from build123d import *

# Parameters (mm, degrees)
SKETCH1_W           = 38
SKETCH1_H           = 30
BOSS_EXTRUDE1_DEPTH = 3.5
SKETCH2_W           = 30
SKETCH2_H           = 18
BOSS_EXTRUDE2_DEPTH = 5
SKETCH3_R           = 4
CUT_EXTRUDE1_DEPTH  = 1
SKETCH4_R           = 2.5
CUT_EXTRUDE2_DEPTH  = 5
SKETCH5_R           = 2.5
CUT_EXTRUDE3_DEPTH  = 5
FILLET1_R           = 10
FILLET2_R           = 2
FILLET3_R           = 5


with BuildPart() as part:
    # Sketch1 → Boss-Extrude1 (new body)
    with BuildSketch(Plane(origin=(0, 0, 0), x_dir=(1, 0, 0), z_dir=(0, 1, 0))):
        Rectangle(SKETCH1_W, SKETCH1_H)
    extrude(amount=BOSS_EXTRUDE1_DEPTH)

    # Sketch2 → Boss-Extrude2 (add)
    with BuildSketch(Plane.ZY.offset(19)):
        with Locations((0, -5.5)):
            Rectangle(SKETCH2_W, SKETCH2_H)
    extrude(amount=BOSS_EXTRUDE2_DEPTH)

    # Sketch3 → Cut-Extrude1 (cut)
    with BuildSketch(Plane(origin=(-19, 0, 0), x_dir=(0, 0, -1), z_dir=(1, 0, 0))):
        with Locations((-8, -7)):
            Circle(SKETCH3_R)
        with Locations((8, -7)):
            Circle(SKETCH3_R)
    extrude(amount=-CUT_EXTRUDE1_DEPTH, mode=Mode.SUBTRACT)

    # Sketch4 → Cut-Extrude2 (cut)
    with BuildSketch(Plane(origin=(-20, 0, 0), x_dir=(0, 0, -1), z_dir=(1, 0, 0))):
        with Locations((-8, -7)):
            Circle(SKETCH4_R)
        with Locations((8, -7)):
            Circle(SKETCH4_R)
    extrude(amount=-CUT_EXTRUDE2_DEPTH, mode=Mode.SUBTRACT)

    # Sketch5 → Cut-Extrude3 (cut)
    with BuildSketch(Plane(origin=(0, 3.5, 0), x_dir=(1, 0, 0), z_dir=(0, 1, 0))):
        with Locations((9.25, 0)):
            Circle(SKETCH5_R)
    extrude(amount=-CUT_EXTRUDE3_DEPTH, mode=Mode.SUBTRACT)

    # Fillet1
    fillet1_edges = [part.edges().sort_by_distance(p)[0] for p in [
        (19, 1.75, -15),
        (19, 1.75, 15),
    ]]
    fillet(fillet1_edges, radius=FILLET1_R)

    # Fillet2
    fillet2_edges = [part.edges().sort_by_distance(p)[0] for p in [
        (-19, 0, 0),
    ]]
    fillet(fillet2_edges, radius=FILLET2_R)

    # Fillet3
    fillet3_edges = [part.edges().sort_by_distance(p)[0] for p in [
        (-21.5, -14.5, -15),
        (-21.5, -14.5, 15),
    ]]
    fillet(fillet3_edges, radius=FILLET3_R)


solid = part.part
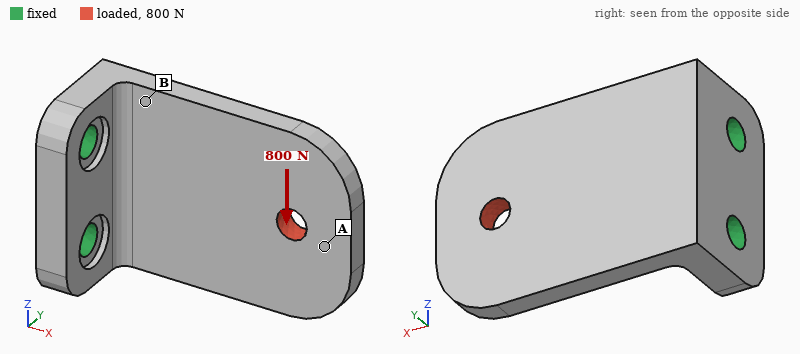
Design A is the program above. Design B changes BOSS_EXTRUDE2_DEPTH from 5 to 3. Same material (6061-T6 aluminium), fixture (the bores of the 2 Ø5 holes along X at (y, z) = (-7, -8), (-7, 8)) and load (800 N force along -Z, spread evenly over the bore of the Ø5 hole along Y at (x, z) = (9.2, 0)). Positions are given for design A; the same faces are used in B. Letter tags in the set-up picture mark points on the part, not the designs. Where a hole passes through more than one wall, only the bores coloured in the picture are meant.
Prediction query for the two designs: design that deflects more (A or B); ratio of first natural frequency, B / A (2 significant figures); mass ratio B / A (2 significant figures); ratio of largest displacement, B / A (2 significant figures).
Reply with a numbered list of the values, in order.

1. B
2. 0.72
3. 0.84
4. 2.3
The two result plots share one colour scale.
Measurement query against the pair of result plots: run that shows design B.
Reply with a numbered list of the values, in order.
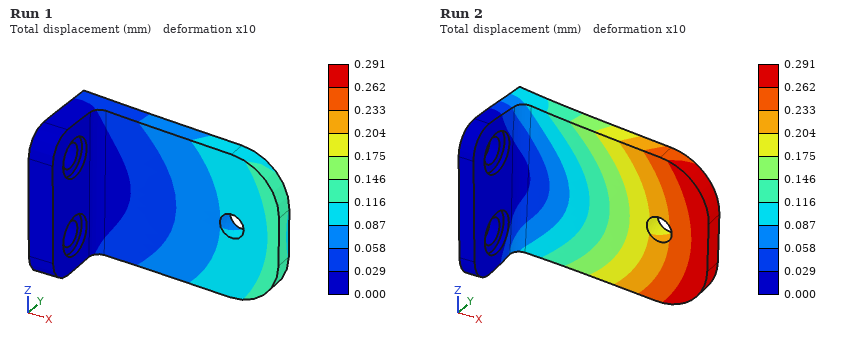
1. Run 2
